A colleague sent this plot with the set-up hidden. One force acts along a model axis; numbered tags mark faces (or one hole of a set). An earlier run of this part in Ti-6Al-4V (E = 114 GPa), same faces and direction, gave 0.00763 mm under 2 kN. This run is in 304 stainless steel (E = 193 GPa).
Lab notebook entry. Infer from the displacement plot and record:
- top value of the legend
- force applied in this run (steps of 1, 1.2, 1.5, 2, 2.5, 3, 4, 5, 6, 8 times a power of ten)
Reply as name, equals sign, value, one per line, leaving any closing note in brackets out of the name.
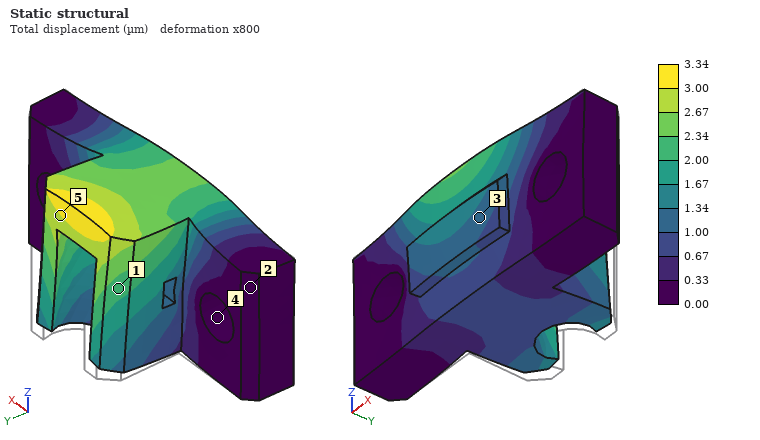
top value of the legend = 3.34 µm
force applied in this run = 1.5 kN
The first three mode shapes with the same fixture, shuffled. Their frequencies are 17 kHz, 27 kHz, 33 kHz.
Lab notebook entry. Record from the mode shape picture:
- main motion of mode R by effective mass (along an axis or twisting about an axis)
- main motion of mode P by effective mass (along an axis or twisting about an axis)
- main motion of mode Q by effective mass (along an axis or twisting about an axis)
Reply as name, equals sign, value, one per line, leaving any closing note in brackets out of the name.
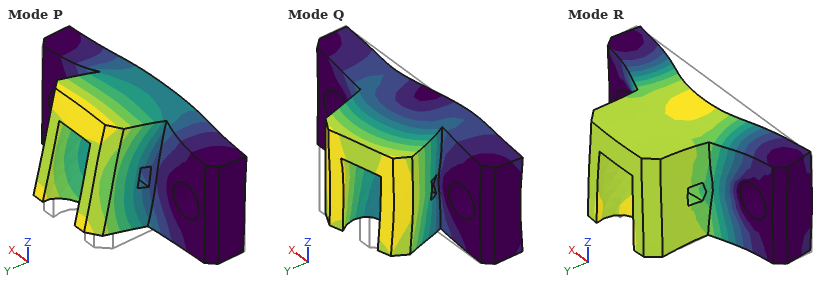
main motion of mode R by effective mass = along Y
main motion of mode P by effective mass = along Z
main motion of mode Q by effective mass = along X
